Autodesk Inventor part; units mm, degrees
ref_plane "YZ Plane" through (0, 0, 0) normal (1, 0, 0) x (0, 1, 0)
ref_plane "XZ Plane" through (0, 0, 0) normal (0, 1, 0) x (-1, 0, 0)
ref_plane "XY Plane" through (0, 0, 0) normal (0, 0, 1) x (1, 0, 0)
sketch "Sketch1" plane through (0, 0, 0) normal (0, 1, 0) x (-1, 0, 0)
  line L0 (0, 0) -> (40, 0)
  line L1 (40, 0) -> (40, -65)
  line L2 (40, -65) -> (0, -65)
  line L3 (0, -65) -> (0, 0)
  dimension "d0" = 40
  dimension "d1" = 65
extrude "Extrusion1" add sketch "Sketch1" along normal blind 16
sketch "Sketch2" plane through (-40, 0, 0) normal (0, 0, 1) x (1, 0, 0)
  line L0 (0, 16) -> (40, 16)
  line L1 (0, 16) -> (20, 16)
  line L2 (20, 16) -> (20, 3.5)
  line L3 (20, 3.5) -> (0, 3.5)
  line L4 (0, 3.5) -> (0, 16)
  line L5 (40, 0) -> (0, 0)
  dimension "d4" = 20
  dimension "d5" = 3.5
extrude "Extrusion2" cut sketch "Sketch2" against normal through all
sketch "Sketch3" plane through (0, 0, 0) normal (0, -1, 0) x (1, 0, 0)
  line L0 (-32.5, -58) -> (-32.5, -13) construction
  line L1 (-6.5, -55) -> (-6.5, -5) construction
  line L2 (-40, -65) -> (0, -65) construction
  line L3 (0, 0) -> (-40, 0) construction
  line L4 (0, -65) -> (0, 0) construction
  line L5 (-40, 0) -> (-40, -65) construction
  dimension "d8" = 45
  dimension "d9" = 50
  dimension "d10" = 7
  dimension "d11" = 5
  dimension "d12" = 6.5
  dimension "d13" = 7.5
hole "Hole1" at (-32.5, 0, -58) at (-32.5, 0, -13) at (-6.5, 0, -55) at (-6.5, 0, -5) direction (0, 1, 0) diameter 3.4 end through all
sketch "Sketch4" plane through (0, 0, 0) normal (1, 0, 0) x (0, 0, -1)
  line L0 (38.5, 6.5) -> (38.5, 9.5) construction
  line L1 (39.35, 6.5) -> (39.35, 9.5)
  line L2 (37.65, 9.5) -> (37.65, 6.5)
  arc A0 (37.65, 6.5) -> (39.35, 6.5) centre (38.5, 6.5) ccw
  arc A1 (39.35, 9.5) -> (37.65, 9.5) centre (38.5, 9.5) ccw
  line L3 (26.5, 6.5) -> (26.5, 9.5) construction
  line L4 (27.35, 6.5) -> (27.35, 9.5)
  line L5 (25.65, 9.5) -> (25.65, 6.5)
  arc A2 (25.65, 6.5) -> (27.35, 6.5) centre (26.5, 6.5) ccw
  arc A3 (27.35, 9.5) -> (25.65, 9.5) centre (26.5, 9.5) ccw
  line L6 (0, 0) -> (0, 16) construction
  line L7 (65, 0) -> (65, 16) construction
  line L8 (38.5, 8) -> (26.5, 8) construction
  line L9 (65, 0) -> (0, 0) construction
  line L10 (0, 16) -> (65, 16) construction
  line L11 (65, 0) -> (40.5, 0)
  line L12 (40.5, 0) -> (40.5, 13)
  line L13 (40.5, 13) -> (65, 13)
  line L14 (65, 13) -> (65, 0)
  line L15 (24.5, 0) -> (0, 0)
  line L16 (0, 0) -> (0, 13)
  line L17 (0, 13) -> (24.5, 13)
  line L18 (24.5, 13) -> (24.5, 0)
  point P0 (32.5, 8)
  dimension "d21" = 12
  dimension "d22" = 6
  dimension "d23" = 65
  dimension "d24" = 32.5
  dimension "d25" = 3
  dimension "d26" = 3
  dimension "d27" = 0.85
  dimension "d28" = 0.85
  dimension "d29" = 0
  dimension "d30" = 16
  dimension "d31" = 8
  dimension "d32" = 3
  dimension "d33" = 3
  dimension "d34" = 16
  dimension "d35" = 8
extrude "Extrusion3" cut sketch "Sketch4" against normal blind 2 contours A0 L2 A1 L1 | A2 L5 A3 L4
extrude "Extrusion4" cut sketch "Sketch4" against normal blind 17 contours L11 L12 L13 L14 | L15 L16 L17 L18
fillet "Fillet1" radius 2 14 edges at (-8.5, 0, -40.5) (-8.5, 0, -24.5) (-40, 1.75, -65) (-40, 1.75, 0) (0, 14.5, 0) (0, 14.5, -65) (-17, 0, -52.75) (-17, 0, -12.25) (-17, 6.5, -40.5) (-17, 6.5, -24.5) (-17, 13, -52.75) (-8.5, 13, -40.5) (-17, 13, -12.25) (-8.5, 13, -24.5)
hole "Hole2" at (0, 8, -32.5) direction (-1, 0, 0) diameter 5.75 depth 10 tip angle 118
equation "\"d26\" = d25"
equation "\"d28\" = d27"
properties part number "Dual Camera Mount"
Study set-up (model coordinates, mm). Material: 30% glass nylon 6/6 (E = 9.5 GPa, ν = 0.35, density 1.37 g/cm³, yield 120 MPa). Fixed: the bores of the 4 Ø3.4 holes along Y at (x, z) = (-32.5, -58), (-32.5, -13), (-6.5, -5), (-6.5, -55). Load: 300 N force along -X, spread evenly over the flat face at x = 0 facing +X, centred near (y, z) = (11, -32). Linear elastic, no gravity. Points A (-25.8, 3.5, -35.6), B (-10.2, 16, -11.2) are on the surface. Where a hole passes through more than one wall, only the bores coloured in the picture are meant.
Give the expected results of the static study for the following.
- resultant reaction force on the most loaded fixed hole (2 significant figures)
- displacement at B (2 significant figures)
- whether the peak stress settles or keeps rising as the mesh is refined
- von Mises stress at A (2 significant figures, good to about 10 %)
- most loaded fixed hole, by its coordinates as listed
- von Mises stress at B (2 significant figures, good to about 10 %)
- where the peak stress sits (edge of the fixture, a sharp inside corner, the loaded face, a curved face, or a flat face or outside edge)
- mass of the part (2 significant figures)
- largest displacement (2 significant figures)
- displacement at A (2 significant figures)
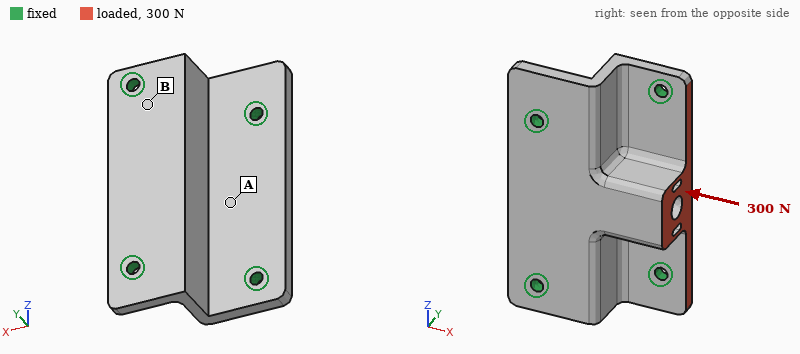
110 N
5.0 µm
keeps rising
0.87 MPa
(-6.5, -55)
2.8 MPa
edge of the fixture
19 g
16 µm
6.2 µm
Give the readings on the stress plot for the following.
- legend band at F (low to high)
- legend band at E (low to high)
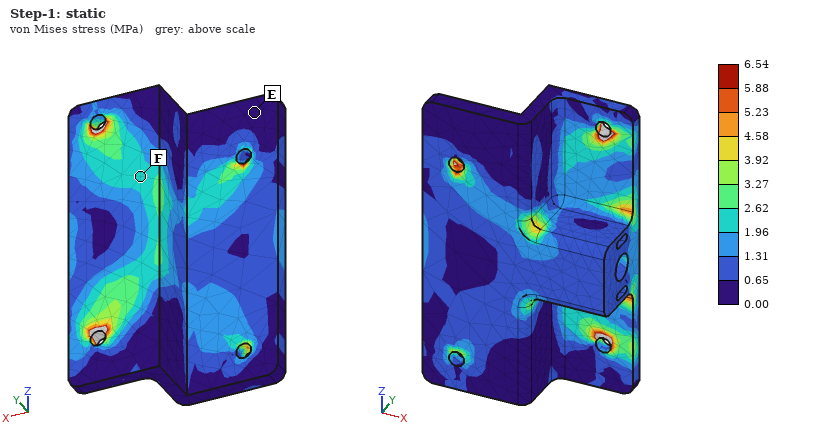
1.96 to 2.62 MPa
0.00 to 0.65 MPa
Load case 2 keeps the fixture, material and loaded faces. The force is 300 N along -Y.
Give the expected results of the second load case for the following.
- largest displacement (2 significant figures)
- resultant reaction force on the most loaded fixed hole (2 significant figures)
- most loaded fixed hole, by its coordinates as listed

0.10 mm
190 N
(-6.5, -55)
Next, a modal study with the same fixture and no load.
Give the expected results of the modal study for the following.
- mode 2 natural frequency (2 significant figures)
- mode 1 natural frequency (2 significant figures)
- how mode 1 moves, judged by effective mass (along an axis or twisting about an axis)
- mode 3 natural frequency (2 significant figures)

5900 Hz
3500 Hz
along Y
7100 Hz
